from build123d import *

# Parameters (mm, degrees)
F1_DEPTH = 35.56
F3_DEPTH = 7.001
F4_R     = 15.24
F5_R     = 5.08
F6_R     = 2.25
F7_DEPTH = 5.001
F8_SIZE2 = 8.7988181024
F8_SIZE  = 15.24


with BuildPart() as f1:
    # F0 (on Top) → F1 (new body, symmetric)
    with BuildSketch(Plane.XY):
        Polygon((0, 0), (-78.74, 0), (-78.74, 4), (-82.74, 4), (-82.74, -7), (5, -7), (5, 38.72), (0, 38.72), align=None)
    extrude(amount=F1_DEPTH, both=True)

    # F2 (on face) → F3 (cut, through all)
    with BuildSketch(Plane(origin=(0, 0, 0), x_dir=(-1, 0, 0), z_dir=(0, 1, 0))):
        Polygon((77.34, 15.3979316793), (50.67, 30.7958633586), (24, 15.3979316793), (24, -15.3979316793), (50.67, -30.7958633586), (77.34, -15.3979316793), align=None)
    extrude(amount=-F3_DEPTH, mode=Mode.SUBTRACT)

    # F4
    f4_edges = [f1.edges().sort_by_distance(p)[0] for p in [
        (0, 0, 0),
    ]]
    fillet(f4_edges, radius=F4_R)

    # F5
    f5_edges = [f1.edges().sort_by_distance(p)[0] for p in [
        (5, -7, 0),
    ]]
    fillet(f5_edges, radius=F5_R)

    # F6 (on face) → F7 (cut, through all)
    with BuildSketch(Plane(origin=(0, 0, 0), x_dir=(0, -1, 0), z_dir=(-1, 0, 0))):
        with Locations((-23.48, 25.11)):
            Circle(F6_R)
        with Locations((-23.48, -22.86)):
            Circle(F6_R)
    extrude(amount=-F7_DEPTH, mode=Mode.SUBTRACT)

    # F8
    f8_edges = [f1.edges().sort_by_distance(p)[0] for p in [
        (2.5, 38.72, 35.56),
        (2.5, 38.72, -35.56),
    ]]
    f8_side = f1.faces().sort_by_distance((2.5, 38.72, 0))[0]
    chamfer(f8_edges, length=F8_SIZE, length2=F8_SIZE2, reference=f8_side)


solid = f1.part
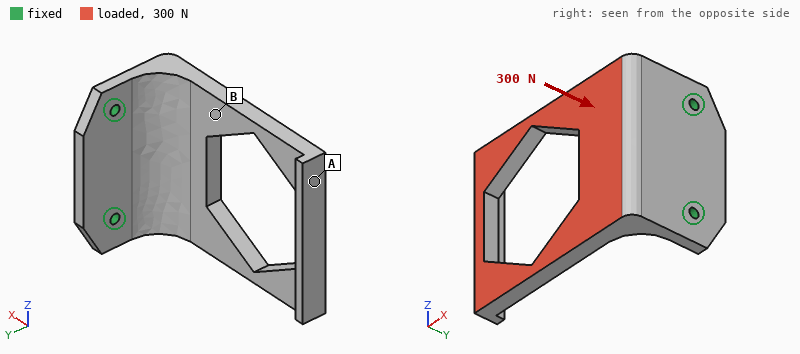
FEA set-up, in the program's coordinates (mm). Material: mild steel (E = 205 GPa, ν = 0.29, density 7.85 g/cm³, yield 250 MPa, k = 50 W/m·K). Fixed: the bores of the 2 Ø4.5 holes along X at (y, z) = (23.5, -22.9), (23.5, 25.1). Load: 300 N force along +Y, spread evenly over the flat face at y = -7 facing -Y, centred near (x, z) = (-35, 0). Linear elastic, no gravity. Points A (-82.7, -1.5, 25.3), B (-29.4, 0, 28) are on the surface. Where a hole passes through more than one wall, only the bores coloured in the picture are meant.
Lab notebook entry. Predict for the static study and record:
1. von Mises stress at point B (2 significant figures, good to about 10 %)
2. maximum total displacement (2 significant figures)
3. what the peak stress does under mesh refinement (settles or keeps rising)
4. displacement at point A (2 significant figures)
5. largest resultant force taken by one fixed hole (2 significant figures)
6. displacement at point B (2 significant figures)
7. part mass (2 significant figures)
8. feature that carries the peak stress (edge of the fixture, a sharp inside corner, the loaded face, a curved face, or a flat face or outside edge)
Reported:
17 MPa
0.18 mm
keeps rising
0.18 mm
160 N
0.051 mm
340 g
edge of the fixture
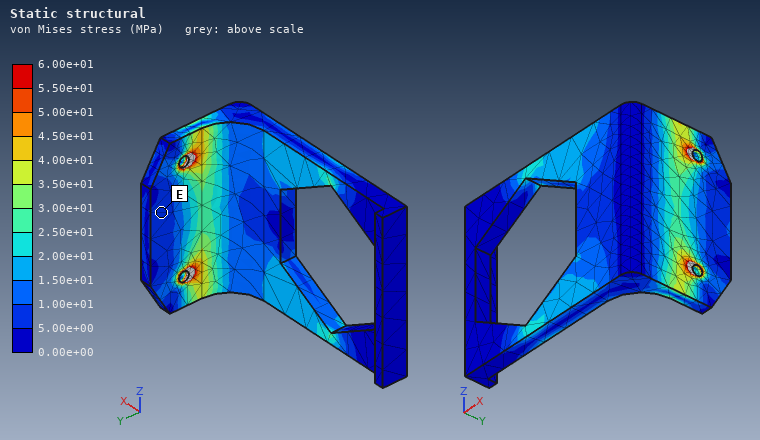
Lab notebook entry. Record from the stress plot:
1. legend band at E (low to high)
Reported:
5.00e+00 to 1.00e+01 MPa
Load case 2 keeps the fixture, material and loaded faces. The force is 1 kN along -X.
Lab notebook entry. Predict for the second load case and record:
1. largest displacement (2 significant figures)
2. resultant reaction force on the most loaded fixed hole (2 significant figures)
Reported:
0.27 mm
520 N
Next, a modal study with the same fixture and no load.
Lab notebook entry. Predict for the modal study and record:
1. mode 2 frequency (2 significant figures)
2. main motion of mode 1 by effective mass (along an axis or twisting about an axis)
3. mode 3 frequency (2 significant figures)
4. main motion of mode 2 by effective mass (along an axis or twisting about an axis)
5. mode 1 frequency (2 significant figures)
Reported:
1300 Hz
along Y
1800 Hz
along Z
520 Hz
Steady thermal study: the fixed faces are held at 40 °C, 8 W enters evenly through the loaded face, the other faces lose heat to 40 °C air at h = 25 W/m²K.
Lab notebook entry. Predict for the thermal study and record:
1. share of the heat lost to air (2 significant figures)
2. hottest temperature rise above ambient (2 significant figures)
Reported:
38 %
19 K
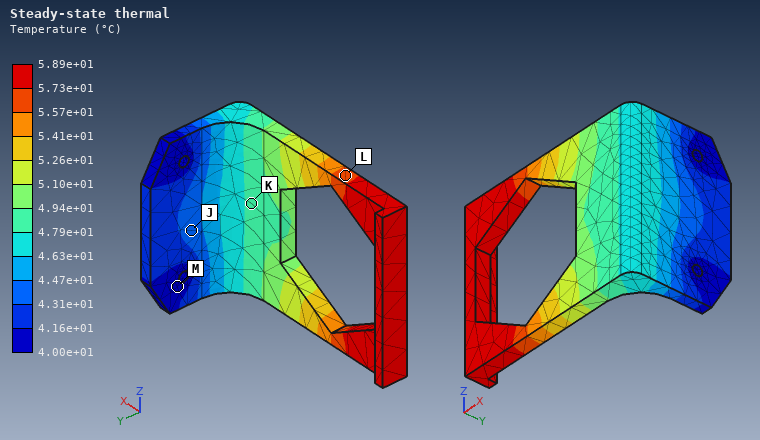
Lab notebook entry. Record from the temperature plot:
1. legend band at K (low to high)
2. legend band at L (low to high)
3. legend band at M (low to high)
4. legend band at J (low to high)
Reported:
4.79e+01 to 4.94e+01 °C
5.57e+01 to 5.73e+01 °C
4.00e+01 to 4.16e+01 °C
4.31e+01 to 4.47e+01 °C
